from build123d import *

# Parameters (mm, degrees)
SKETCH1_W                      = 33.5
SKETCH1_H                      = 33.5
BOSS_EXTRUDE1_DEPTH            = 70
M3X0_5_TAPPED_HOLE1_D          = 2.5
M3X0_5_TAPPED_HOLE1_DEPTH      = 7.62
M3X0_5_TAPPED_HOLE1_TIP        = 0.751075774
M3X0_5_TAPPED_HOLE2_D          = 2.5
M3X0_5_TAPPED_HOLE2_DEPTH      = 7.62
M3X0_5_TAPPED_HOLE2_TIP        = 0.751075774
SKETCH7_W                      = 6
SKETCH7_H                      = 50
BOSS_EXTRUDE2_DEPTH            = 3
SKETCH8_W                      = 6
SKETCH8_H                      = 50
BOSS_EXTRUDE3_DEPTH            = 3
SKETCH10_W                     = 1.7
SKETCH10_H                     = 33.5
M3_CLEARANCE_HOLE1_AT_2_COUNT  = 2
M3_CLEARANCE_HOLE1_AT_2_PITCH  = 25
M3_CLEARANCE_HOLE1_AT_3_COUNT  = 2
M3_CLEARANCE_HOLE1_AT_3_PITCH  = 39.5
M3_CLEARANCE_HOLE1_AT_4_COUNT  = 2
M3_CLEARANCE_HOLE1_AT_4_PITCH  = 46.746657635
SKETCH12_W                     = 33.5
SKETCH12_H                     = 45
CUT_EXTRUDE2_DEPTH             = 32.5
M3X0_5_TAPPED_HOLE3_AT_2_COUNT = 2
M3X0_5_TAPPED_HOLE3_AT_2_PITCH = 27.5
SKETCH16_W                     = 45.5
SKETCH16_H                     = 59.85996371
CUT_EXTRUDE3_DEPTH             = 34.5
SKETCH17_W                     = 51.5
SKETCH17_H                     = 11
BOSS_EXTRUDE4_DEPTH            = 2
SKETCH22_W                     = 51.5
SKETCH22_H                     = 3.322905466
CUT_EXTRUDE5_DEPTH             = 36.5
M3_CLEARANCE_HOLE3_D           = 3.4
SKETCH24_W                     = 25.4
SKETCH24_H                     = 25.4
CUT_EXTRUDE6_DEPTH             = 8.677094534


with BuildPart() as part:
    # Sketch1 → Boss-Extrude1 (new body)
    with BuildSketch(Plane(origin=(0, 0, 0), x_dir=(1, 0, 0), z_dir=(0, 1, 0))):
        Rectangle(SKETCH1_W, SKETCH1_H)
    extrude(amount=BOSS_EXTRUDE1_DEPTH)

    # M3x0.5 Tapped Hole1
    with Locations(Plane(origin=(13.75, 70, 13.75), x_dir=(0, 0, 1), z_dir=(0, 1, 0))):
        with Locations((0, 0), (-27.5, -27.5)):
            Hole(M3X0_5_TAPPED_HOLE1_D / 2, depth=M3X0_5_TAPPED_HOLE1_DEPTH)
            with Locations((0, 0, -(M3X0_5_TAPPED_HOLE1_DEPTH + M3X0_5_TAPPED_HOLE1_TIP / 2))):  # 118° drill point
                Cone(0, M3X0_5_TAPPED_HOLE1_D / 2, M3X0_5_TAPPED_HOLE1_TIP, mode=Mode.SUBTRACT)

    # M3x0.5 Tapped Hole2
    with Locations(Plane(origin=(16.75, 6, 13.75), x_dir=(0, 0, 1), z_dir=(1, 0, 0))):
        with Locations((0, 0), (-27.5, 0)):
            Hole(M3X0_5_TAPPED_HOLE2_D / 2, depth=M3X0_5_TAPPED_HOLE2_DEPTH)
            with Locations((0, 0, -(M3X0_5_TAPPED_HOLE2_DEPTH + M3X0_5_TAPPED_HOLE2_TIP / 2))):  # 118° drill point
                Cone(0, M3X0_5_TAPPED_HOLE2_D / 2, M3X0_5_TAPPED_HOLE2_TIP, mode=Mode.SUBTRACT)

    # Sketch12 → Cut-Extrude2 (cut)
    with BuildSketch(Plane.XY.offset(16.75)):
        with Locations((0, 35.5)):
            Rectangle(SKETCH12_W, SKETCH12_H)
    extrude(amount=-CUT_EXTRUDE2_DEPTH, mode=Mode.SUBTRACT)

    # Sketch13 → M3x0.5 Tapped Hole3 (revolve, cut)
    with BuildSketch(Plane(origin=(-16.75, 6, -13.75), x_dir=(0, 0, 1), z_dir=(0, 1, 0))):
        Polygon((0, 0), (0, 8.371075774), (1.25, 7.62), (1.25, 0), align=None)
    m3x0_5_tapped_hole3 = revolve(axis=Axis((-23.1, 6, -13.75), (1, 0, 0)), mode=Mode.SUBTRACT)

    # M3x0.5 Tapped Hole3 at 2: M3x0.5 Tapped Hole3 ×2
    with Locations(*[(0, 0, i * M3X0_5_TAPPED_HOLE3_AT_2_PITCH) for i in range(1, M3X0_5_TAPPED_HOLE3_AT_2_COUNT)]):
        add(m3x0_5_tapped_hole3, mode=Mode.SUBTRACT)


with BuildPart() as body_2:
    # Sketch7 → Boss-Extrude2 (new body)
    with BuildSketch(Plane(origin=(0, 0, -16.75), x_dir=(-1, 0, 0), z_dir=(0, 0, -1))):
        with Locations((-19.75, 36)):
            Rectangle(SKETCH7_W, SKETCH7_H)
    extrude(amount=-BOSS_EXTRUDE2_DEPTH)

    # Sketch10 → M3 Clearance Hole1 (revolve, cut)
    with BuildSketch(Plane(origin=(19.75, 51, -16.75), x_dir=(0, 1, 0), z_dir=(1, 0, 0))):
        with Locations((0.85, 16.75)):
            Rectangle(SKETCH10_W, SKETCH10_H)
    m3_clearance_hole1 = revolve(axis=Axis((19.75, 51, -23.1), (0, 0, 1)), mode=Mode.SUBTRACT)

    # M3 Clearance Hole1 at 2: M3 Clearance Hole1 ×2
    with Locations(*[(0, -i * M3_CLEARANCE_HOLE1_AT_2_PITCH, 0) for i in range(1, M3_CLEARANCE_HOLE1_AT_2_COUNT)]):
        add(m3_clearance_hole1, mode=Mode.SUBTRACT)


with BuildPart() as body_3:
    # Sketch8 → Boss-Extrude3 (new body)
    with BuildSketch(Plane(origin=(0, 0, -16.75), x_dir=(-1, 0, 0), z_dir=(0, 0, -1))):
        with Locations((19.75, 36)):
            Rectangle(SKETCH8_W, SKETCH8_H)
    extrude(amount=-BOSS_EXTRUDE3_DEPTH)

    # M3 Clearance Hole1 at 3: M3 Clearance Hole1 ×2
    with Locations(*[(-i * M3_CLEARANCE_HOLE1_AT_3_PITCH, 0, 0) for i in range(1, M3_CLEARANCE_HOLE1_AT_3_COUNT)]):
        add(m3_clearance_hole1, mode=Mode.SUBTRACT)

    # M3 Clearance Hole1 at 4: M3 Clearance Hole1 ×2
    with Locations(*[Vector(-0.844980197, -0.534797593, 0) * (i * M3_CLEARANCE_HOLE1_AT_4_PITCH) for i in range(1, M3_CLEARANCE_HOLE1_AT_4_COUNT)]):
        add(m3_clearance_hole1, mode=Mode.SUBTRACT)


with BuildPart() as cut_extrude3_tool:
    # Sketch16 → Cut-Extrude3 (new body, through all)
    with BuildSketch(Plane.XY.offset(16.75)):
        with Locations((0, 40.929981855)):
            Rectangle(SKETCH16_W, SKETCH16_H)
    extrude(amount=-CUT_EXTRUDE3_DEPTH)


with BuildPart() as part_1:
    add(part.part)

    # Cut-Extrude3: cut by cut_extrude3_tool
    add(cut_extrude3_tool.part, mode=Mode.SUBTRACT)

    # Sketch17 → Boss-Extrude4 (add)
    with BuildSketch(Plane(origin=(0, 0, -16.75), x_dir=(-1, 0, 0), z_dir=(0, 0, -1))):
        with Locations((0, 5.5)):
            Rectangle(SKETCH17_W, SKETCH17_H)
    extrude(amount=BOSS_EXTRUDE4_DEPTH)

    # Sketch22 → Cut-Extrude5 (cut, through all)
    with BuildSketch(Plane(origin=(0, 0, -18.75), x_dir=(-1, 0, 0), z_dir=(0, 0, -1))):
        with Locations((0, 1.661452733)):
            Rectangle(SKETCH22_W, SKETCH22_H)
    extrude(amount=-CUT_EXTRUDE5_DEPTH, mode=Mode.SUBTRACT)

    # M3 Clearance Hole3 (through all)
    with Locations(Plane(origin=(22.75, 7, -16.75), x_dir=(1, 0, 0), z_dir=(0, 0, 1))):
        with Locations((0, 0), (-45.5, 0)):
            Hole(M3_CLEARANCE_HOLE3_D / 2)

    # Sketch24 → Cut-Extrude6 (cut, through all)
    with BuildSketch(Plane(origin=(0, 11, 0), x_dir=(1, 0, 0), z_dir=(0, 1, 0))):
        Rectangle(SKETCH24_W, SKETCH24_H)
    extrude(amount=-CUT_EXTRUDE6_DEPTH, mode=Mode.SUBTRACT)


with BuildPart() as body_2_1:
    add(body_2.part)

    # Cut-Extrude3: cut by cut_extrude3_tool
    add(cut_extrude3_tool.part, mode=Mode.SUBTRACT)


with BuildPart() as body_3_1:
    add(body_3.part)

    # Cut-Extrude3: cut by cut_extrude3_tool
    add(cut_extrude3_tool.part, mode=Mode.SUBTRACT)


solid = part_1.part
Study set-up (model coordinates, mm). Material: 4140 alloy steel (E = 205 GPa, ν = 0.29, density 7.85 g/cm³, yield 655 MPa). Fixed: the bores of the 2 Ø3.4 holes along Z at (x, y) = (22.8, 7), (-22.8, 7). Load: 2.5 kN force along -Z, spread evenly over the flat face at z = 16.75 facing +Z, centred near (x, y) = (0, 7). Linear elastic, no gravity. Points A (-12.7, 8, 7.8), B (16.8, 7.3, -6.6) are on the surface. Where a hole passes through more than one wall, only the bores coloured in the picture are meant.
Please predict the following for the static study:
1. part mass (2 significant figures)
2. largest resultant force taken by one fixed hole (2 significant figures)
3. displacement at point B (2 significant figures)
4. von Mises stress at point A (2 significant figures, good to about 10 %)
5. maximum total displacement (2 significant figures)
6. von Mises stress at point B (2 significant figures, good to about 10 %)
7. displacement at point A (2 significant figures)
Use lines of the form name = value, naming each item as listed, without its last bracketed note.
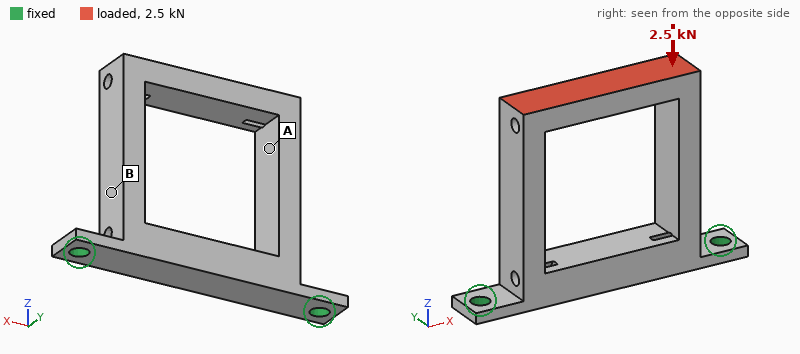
part mass = 33 g
largest resultant force taken by one fixed hole = 1.4 kN
displacement at point B = 34 µm
von Mises stress at point A = 150 MPa
maximum total displacement = 76 µm
von Mises stress at point B = 64 MPa
displacement at point A = 38 µm
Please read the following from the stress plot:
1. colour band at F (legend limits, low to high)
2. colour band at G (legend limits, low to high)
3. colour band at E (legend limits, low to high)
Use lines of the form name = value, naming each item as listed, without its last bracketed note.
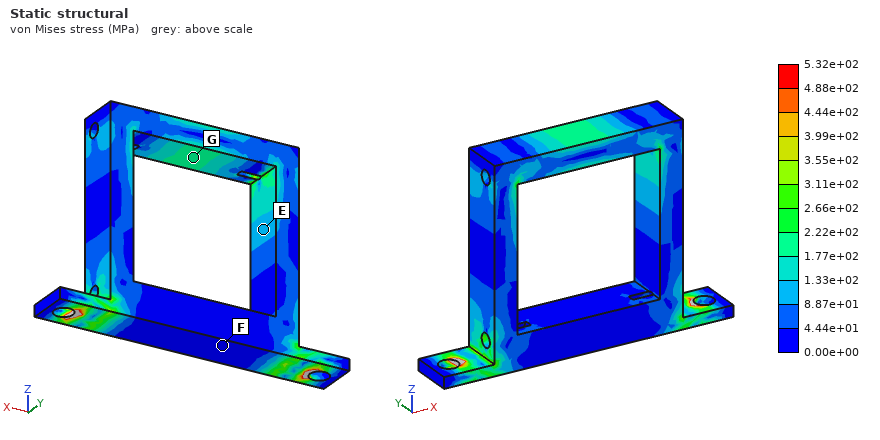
colour band at F = 0.00e+00 to 4.44e+01 MPa
colour band at G = 1.77e+02 to 2.22e+02 MPa
colour band at E = 8.87e+01 to 1.33e+02 MPa
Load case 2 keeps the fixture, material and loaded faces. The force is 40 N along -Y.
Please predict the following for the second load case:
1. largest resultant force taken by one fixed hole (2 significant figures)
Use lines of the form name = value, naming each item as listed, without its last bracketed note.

largest resultant force taken by one fixed hole = 20 N
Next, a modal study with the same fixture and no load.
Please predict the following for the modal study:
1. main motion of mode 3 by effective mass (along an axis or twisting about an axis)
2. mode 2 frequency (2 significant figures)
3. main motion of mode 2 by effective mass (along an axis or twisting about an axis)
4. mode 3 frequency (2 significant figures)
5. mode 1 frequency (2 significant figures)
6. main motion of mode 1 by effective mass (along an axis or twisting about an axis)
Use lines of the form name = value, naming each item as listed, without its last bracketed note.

main motion of mode 3 by effective mass = twisting about Z
mode 2 frequency = 3000 Hz
main motion of mode 2 by effective mass = along X
mode 3 frequency = 4700 Hz
mode 1 frequency = 1100 Hz
main motion of mode 1 by effective mass = along Y
